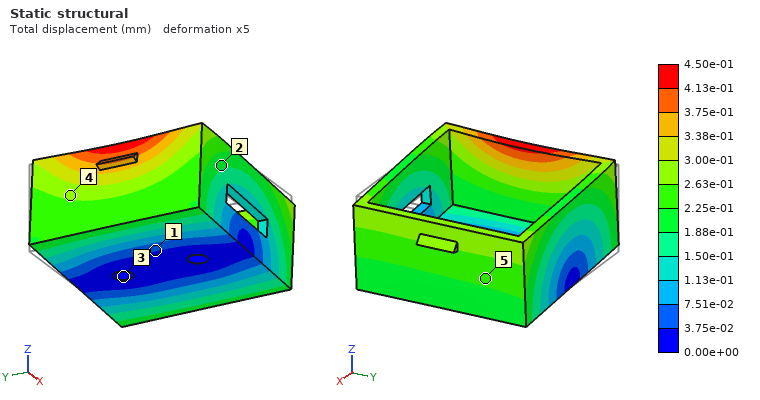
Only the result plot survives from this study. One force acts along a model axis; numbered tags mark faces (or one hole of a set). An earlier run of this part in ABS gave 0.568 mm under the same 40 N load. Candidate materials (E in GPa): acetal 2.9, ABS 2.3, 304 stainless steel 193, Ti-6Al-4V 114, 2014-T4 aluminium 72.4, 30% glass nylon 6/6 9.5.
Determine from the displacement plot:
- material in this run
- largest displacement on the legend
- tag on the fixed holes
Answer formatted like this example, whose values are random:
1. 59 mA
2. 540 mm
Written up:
1. acetal
2. 4.50e-01 mm
3. 3
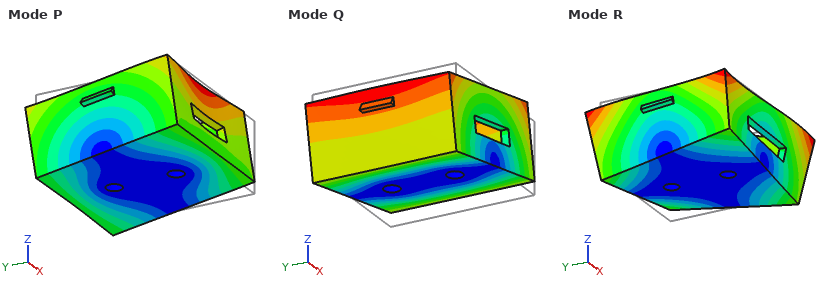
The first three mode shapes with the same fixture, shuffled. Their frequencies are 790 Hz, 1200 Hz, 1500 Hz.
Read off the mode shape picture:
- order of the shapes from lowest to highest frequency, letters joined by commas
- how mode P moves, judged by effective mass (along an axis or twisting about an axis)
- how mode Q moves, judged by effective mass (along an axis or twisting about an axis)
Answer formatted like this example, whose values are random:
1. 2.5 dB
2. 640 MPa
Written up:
1. Q, R, P
2. along Y
3. along X
